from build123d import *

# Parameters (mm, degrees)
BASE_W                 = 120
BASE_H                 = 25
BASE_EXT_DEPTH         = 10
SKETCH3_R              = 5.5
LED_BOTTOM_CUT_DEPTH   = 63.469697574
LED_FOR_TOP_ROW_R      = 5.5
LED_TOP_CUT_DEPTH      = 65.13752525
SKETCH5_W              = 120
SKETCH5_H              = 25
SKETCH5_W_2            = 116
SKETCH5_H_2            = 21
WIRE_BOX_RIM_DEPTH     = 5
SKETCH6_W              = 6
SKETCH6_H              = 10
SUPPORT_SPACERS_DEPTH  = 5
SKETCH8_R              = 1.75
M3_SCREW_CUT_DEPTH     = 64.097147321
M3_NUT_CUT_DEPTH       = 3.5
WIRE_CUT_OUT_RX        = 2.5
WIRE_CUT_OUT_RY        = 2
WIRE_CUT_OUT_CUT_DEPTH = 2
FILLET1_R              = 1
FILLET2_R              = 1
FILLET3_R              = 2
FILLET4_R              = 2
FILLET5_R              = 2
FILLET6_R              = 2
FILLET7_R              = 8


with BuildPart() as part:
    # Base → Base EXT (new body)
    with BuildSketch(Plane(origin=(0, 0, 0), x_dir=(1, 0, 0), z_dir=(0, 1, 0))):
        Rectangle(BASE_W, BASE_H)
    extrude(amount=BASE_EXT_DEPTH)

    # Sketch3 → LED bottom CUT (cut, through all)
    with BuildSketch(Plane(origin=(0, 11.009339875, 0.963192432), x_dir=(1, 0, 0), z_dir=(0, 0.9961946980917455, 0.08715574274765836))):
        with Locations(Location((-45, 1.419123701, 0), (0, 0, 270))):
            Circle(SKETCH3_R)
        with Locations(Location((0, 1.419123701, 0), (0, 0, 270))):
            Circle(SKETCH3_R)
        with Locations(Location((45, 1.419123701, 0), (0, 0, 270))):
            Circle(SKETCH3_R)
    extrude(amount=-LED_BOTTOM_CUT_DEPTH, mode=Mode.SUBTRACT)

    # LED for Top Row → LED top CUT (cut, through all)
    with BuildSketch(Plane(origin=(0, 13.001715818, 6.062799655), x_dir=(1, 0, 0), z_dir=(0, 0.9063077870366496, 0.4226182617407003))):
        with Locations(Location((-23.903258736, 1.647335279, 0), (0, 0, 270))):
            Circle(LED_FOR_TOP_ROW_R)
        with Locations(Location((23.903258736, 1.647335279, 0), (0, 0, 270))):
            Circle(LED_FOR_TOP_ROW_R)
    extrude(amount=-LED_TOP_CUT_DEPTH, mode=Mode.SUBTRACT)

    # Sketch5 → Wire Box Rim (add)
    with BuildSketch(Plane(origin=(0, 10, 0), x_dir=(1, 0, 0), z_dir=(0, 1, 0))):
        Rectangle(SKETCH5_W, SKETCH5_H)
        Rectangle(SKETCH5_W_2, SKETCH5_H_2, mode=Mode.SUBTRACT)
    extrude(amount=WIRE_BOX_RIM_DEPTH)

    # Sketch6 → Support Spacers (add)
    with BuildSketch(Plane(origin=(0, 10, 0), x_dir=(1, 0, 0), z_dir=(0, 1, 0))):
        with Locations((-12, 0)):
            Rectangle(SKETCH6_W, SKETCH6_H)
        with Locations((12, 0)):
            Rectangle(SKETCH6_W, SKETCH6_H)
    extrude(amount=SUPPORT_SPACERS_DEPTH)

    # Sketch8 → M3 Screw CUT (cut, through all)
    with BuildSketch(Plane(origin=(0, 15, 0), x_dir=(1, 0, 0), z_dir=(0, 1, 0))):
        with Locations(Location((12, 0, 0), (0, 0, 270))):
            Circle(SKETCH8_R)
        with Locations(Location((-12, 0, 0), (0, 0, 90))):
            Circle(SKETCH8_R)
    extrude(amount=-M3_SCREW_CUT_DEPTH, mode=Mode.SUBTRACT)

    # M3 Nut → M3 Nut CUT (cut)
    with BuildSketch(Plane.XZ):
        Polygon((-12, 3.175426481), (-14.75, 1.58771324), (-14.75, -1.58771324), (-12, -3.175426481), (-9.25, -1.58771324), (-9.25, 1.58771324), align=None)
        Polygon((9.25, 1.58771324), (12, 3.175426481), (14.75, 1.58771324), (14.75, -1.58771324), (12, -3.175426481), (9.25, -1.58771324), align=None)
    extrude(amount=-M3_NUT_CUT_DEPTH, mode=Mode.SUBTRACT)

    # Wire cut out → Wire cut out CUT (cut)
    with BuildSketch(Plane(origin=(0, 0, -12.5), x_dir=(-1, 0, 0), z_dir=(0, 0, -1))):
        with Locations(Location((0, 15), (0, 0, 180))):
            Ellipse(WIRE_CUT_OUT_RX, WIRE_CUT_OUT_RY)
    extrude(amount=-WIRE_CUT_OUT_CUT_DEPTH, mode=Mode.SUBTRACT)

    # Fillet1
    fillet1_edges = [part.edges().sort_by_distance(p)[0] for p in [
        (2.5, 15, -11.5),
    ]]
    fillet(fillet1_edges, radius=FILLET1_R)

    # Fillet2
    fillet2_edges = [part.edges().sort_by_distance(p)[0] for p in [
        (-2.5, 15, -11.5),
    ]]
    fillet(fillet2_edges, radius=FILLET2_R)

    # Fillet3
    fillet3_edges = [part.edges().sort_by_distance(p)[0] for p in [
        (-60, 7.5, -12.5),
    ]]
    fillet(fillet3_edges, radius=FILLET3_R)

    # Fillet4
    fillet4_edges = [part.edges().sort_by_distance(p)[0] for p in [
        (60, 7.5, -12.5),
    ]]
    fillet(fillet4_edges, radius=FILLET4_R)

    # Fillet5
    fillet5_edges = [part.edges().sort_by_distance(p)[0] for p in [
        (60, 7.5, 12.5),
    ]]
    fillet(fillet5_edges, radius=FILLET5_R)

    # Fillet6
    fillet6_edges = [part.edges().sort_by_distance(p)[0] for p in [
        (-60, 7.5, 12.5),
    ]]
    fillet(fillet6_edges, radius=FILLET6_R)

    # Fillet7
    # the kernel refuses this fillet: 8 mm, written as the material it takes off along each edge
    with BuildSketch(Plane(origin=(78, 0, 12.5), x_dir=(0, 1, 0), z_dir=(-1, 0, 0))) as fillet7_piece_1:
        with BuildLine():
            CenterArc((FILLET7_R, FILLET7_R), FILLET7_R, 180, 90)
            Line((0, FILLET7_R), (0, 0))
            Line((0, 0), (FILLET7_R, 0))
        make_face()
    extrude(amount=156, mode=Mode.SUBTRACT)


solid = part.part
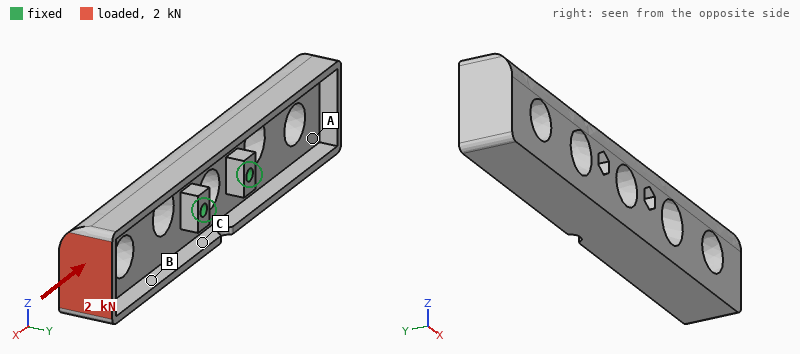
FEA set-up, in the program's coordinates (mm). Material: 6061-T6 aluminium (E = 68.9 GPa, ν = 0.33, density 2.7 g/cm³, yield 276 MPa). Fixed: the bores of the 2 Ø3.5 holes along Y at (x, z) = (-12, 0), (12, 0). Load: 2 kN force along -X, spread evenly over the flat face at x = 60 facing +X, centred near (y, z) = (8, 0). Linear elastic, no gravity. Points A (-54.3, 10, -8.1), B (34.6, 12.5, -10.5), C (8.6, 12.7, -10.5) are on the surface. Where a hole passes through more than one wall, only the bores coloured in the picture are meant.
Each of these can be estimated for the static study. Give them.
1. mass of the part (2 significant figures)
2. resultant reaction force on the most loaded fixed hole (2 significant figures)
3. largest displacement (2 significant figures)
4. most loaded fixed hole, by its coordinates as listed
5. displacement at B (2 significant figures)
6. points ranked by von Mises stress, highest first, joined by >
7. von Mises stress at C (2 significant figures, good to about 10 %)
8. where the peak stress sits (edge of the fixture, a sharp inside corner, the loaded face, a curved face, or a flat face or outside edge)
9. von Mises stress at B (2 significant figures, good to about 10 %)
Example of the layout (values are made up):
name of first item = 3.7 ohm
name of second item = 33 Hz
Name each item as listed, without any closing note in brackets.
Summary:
mass of the part = 71 g
resultant reaction force on the most loaded fixed hole = 1.4 kN
largest displacement = 54 µm
most loaded fixed hole, by its coordinates as listed = (12, 0)
displacement at B = 11 µm
points ranked by von Mises stress, highest first, joined by > = B > C > A
von Mises stress at C = 9.7 MPa
where the peak stress sits = the loaded face
von Mises stress at B = 19 MPa
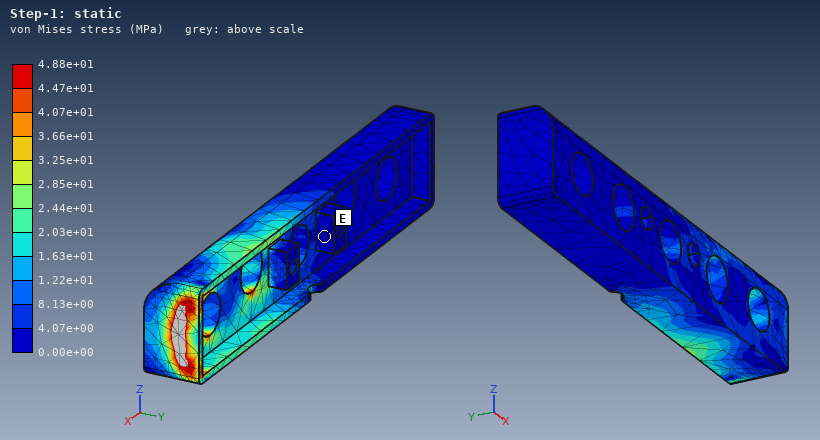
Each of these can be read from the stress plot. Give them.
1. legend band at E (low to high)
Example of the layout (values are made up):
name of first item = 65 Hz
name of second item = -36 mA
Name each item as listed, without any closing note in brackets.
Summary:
legend band at E = 0.00e+00 to 4.07e+00 MPa
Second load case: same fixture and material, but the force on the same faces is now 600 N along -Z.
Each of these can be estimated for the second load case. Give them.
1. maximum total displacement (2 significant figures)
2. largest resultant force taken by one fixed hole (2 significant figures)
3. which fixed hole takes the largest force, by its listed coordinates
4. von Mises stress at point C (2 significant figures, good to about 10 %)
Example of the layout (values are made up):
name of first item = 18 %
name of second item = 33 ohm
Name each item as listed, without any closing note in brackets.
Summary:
maximum total displacement = 83 µm
largest resultant force taken by one fixed hole = 1.5 kN
which fixed hole takes the largest force, by its listed coordinates = (12, 0)
von Mises stress at point C = 12 MPa
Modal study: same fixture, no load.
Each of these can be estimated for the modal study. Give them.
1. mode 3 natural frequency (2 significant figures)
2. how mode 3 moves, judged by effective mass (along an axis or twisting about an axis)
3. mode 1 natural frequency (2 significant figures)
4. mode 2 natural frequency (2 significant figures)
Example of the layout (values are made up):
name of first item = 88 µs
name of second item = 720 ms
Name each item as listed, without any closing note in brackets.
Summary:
mode 3 natural frequency = 4200 Hz
how mode 3 moves, judged by effective mass = twisting about Y
mode 1 natural frequency = 2900 Hz
mode 2 natural frequency = 2900 Hz
